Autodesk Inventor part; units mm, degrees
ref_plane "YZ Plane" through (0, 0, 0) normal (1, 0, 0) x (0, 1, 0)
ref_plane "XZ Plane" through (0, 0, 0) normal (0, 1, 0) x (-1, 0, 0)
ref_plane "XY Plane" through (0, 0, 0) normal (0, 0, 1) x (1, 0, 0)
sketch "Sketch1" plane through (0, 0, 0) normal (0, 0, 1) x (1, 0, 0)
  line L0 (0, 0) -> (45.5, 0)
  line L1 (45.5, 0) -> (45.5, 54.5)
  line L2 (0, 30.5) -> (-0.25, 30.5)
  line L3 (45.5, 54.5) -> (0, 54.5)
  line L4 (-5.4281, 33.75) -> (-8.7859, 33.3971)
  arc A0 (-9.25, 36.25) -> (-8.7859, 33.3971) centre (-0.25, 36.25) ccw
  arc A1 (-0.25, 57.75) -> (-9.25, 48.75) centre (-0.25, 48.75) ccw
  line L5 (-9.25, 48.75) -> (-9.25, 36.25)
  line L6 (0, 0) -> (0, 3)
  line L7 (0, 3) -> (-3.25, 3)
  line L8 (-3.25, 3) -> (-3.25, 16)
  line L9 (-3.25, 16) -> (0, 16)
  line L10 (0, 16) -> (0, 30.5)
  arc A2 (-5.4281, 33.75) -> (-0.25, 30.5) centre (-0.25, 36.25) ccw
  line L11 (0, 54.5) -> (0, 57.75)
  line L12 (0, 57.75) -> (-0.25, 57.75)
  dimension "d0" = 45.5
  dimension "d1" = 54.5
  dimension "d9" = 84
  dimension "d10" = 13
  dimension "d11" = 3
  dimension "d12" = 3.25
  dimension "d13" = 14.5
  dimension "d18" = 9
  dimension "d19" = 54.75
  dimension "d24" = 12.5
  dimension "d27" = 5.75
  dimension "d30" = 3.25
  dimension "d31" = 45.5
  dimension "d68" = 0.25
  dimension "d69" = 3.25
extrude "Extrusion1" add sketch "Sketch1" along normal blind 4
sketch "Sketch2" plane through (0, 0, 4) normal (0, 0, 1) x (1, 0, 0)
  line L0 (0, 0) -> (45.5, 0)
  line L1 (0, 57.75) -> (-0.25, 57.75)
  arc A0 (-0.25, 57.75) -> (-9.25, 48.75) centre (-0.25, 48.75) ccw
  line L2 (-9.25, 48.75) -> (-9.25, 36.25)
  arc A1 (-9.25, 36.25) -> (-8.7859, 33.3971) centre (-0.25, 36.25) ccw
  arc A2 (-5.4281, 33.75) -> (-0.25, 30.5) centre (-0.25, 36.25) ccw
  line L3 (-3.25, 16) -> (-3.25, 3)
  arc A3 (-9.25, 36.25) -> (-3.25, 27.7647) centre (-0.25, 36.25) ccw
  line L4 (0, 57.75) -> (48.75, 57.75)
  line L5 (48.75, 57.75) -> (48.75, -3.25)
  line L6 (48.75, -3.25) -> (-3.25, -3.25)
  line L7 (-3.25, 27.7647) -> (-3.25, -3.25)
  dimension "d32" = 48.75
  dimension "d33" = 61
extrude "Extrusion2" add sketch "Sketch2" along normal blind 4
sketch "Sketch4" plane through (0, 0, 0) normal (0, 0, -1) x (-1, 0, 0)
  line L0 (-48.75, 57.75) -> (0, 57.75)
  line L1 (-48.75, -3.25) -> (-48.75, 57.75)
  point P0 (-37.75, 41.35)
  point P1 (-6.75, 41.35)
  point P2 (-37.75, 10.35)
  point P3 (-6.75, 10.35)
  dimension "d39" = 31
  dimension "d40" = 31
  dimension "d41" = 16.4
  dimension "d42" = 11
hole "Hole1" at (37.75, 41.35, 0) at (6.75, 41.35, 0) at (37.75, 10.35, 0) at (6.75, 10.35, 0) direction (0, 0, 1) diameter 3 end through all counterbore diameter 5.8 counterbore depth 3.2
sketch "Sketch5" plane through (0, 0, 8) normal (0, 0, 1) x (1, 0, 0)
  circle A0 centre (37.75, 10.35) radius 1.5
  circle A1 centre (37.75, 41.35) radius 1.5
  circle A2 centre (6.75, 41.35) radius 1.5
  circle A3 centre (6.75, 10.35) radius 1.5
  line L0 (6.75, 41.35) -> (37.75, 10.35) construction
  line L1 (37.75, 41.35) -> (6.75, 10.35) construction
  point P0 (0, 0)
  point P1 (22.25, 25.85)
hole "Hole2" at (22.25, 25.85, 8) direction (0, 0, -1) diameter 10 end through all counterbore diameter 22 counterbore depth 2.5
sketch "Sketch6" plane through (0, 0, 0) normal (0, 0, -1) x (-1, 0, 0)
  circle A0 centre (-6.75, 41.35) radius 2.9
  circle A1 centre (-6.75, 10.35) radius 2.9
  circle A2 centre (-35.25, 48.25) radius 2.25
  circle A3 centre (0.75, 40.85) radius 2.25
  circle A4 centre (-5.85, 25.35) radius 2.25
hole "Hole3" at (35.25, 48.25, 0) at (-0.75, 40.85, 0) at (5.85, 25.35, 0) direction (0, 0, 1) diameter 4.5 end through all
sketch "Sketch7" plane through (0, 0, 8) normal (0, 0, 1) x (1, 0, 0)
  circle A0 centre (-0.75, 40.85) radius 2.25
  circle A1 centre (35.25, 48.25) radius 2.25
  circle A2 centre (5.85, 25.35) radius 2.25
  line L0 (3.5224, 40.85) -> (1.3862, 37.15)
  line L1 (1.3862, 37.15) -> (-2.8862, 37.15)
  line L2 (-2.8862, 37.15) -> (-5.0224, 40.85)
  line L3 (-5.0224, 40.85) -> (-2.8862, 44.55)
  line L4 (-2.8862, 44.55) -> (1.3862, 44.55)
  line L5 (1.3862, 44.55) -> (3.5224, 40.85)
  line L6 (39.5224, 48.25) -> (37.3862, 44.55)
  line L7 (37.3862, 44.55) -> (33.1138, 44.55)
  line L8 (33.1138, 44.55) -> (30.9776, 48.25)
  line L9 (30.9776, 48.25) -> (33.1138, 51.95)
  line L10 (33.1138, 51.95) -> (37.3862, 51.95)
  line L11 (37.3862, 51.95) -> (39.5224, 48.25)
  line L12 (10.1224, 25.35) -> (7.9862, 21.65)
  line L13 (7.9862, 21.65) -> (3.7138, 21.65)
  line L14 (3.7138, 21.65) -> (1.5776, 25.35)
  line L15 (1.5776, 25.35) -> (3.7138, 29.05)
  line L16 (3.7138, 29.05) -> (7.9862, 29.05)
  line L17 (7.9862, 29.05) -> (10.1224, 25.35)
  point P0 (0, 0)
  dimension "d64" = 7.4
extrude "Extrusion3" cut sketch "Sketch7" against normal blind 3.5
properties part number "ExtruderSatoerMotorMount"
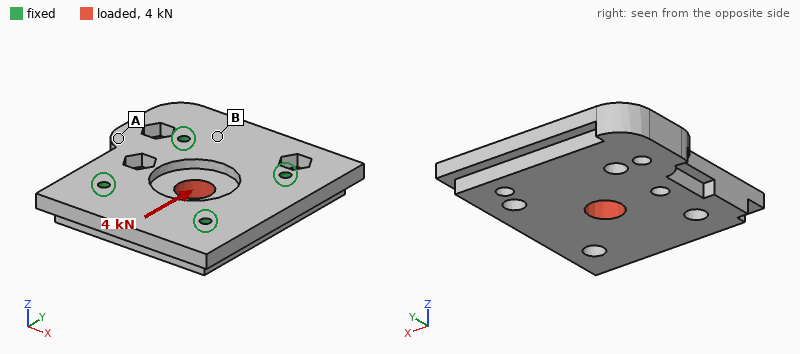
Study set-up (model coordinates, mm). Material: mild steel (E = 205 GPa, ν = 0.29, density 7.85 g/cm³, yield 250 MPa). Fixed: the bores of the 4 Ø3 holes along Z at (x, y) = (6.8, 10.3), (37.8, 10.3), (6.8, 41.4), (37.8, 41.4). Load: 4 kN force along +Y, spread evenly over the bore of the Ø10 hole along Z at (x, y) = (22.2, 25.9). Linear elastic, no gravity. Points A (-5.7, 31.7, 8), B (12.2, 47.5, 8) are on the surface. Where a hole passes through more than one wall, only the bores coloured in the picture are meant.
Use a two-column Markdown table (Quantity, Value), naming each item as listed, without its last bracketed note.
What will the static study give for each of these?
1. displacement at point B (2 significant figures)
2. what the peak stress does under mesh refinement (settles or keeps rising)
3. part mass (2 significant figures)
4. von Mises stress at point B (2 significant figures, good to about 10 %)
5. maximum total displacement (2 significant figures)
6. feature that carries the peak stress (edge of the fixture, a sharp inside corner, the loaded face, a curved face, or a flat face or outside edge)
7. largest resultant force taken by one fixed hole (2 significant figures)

| Quantity | Value |
|---|---|
| displacement at point B | 0.57 µm |
| what the peak stress does under mesh refinement | keeps rising |
| part mass | 170 g |
| von Mises stress at point B | 7.3 MPa |
| maximum total displacement | 2.1 µm |
| feature that carries the peak stress | edge of the fixture |
| largest resultant force taken by one fixed hole | 1.1 kN |
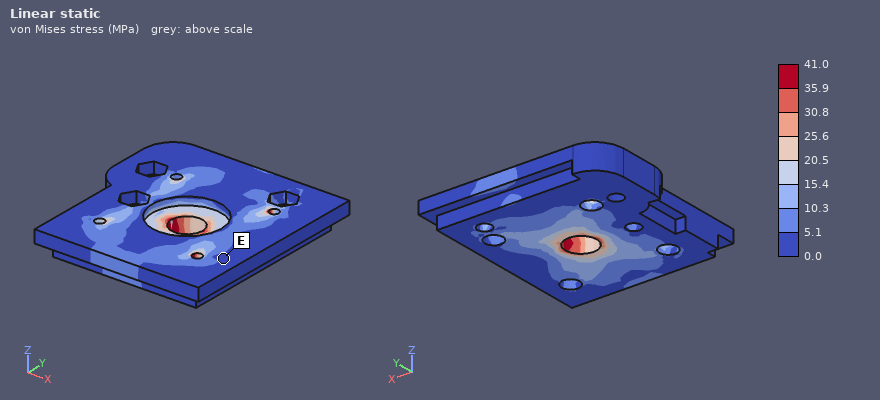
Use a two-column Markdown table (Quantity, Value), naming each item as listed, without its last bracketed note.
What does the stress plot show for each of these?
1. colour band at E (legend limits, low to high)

| Quantity | Value |
|---|---|
| colour band at E | 0.0 to 5.1 MPa |
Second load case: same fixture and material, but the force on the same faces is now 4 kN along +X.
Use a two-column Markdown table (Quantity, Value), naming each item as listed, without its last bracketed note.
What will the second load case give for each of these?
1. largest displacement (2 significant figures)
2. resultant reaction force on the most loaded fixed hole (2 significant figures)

| Quantity | Value |
|---|---|
| largest displacement | 2.2 µm |
| resultant reaction force on the most loaded fixed hole | 1.1 kN |
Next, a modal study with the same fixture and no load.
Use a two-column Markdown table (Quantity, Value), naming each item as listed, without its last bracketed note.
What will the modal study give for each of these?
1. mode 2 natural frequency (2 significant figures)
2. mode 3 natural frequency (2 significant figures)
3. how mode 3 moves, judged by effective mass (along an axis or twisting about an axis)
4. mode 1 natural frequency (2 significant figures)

| Quantity | Value |
|---|---|
| mode 2 natural frequency | 14 kHz |
| mode 3 natural frequency | 18 kHz |
| how mode 3 moves, judged by effective mass | twisting about X |
| mode 1 natural frequency | 13 kHz |
